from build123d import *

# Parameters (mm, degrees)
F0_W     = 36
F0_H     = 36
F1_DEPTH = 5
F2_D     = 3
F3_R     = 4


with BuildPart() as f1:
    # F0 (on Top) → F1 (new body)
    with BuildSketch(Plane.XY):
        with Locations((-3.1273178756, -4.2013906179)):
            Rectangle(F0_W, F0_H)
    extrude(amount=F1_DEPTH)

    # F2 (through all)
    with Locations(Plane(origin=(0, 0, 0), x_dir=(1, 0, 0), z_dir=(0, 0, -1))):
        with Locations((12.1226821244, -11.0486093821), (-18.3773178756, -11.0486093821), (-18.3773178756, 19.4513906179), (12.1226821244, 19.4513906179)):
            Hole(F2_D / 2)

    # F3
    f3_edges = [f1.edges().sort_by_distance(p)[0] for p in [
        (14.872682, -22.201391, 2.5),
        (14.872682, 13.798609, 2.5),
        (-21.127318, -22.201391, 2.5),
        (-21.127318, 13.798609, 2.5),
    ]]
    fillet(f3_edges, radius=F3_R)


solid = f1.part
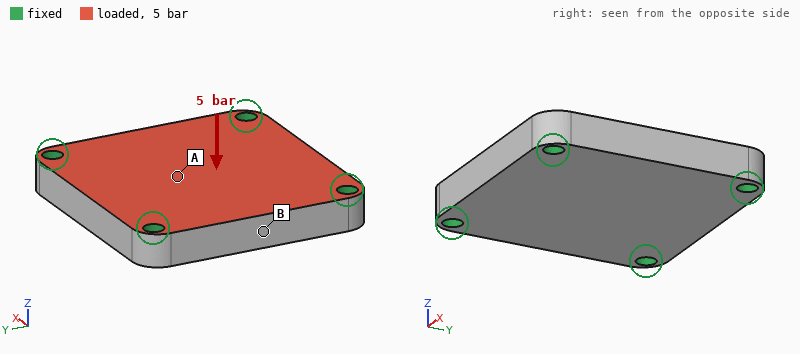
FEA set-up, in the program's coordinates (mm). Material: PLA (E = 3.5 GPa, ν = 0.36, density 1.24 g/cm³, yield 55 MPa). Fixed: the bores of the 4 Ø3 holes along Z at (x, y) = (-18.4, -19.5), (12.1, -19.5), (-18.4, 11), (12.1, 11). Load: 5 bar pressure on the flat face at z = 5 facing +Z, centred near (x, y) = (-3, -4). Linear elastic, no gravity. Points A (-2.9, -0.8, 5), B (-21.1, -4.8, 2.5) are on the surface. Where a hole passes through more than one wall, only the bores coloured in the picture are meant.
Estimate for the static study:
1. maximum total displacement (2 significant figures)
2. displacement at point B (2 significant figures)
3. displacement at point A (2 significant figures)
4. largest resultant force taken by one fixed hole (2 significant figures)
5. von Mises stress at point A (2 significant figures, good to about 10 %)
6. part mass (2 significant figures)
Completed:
94 µm
48 µm
91 µm
160 N
5.7 MPa
7.8 g
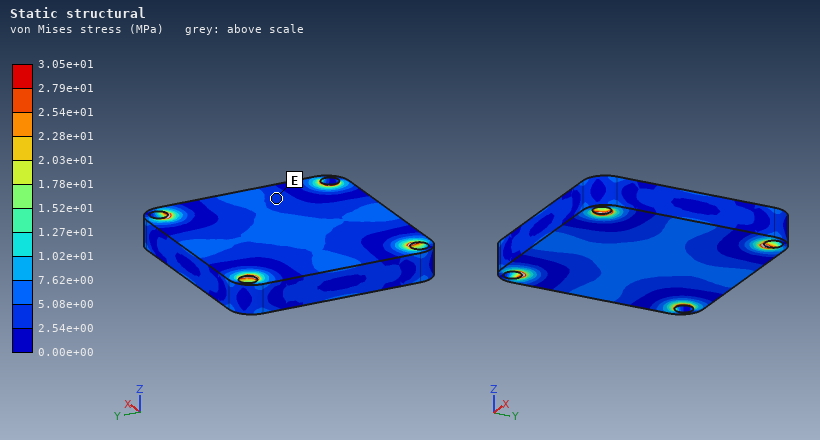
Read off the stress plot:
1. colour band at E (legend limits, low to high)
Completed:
2.54e+00 to 5.08e+00 MPa
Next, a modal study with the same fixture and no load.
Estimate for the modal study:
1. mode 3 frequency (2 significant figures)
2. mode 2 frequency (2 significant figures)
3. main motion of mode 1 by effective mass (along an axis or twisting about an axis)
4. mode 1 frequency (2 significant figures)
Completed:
9000 Hz
9000 Hz
along Z
5500 Hz
